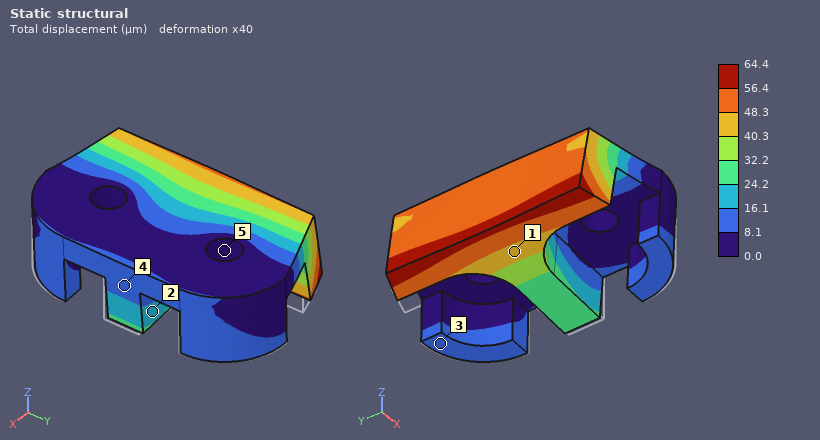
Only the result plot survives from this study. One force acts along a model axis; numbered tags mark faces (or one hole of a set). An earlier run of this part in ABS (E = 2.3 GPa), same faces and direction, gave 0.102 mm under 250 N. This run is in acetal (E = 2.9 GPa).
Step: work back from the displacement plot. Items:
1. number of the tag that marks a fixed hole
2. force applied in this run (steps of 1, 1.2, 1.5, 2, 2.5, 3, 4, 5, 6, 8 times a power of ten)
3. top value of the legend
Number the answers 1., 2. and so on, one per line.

1. 5
2. 200 N
3. 64.4 µm
